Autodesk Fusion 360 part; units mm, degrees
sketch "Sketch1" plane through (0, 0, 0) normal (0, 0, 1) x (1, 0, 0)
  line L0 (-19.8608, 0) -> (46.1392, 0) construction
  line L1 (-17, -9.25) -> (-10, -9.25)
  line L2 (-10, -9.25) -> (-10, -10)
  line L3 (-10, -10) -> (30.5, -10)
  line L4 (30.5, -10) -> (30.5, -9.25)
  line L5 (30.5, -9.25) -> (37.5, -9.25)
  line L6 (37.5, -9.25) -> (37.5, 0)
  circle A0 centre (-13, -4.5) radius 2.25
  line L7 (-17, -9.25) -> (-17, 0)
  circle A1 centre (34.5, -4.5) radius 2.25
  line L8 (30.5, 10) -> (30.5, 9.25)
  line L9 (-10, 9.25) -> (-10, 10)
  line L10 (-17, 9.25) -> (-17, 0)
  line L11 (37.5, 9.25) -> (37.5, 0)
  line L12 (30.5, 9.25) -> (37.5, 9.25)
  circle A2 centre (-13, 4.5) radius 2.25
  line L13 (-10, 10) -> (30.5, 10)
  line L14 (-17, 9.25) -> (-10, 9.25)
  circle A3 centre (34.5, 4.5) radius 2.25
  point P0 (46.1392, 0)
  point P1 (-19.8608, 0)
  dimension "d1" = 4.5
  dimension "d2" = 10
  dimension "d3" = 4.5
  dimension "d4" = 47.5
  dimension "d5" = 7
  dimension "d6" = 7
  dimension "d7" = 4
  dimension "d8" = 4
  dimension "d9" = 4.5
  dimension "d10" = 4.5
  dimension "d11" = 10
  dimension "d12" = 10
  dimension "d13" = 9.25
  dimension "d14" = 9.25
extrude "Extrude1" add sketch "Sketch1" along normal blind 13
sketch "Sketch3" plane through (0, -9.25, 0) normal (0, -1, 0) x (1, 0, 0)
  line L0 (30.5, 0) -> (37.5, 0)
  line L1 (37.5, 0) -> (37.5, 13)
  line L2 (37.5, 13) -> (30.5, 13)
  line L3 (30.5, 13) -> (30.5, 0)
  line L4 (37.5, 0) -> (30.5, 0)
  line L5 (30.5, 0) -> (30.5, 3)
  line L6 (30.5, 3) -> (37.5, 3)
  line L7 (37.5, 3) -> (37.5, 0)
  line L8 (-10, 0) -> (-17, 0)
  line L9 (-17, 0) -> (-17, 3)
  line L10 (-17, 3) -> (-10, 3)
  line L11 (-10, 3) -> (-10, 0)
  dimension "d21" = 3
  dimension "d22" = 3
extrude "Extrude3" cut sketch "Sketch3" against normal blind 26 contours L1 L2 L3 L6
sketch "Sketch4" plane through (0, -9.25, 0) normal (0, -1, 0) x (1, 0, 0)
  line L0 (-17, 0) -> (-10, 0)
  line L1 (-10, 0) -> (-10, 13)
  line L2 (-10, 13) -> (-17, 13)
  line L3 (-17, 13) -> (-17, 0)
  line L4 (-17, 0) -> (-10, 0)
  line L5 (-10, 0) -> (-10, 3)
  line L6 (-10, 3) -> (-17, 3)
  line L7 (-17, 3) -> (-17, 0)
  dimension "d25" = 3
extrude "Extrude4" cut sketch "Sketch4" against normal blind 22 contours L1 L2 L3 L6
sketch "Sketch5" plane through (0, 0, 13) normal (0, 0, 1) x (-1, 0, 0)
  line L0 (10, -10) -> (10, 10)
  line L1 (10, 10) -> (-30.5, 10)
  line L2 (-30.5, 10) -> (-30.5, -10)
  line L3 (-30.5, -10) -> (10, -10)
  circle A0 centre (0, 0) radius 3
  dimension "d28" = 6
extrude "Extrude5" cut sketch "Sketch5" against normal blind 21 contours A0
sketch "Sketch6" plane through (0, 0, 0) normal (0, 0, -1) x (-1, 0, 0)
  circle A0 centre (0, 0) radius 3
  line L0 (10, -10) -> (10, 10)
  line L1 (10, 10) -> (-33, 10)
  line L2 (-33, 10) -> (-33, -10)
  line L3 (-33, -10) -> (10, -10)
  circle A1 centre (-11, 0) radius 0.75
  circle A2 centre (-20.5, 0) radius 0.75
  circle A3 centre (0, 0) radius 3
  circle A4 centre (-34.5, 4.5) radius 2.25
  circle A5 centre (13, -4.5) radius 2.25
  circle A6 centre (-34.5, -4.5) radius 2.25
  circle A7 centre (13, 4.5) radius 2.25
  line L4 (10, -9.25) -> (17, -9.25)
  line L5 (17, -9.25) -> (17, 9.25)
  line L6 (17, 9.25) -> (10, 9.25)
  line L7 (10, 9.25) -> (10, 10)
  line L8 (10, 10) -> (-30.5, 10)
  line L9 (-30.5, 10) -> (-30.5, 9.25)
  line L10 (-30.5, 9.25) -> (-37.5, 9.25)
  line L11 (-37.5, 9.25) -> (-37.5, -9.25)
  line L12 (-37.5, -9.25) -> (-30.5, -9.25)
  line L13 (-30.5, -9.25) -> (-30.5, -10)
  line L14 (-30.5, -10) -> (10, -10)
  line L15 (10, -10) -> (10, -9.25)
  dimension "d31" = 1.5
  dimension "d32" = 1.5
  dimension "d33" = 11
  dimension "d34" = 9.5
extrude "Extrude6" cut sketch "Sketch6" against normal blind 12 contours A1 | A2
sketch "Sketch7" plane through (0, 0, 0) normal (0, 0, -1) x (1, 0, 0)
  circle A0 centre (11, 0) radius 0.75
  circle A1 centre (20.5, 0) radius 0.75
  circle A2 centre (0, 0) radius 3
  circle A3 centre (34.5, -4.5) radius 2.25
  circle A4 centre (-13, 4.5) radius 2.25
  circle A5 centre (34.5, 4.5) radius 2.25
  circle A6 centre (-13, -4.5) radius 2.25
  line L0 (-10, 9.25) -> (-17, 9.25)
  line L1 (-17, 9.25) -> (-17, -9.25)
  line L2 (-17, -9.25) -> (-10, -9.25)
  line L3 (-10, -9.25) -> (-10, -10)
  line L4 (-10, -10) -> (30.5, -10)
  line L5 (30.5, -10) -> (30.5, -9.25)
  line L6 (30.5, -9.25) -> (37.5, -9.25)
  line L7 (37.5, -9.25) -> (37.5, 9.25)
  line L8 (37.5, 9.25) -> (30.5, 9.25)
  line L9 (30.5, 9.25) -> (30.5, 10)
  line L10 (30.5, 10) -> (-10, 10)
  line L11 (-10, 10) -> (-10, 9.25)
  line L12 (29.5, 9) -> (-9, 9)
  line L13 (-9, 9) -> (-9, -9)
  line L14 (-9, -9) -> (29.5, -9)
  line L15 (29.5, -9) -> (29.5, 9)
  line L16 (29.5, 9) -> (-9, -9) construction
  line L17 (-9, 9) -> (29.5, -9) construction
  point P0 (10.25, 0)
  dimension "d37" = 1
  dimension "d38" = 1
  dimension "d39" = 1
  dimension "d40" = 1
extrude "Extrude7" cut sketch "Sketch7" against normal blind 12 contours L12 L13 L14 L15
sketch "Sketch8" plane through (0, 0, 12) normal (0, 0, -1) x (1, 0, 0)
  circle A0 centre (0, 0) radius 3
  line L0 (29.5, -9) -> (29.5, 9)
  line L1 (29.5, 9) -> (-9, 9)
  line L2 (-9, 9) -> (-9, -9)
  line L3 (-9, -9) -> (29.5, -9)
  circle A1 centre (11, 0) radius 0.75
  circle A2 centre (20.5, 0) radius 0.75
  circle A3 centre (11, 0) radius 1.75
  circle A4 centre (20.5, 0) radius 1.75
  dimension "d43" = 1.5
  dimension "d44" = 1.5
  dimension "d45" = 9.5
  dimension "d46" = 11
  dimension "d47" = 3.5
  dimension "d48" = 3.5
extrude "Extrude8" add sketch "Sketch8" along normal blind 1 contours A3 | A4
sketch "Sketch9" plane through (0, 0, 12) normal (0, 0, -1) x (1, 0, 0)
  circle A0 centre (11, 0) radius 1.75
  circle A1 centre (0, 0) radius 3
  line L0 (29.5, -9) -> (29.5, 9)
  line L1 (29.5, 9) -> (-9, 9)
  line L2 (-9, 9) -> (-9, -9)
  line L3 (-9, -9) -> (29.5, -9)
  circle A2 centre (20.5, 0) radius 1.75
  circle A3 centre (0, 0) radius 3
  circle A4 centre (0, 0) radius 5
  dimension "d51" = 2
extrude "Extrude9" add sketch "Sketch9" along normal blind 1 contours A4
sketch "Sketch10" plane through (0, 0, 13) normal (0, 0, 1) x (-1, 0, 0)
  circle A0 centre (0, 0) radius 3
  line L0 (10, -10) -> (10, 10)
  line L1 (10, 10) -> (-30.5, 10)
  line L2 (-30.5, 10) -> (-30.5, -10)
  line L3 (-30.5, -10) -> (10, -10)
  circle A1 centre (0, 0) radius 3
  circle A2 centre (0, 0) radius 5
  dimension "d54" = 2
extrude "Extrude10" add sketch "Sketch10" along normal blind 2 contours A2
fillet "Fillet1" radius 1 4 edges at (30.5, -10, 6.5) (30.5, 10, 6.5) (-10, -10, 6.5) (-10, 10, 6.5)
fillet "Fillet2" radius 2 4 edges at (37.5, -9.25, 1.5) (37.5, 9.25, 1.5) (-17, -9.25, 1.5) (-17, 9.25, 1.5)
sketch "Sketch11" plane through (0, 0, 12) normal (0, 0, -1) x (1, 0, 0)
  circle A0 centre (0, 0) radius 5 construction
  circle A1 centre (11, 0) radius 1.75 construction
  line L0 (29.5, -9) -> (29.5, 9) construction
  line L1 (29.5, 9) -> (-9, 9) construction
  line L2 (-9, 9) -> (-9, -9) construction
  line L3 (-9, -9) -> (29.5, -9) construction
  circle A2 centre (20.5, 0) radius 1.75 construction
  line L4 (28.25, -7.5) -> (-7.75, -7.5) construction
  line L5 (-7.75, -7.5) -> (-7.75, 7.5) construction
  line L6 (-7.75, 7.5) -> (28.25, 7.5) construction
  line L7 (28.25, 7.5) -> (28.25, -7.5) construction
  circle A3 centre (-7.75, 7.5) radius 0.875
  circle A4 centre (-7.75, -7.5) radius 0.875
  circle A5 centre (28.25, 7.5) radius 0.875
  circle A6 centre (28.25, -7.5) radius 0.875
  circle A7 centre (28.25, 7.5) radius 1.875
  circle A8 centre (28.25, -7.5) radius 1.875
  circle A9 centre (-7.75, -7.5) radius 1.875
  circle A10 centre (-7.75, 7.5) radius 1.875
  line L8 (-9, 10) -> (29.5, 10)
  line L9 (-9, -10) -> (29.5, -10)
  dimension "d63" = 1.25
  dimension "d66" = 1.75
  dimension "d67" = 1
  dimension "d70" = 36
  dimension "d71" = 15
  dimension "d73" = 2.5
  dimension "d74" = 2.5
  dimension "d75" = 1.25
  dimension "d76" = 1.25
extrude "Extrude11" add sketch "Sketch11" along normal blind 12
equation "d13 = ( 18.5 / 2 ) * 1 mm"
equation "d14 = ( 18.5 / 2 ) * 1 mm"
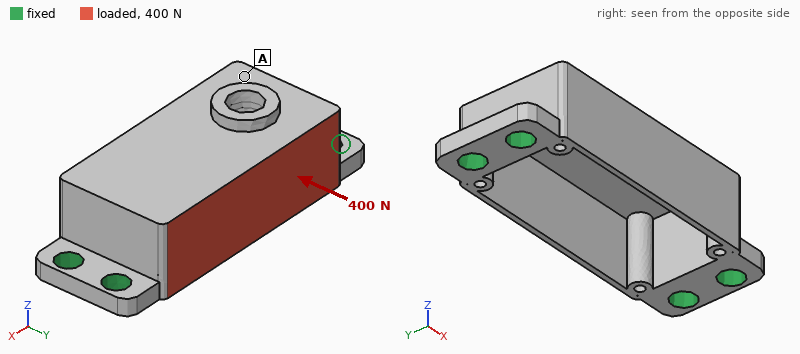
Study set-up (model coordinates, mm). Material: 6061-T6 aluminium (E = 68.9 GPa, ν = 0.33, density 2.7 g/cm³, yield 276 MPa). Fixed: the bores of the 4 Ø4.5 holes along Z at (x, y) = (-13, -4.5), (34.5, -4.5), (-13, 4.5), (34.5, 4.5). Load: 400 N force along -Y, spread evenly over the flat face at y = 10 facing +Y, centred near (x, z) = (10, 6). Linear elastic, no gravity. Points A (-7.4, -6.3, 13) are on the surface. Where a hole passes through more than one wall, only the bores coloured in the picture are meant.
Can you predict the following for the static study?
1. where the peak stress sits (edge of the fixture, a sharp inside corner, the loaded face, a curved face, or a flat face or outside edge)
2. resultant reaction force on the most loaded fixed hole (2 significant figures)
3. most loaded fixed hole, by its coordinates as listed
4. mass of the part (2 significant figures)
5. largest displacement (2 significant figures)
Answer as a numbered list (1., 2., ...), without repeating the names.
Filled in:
1. the loaded face
2. 170 N
3. (-13, 4.5)
4. 8.8 g
5. 0.29 mm
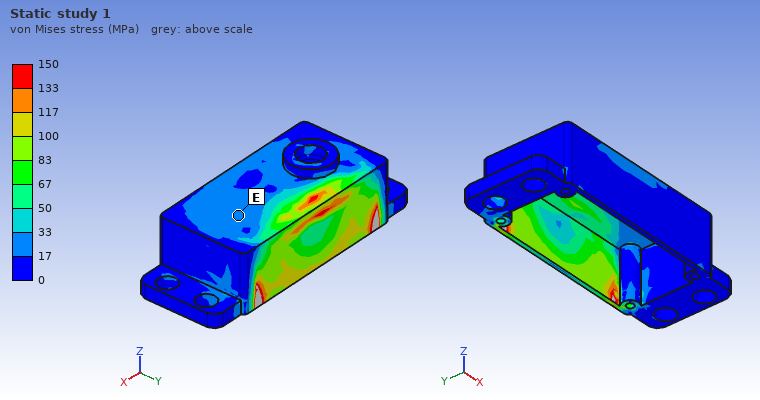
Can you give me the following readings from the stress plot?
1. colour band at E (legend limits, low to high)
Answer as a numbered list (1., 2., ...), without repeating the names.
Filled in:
1. 17 to 33 MPa
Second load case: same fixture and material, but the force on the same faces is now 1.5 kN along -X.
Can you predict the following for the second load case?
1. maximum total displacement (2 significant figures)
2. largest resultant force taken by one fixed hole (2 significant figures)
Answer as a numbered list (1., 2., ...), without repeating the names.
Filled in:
1. 35 µm
2. 640 N
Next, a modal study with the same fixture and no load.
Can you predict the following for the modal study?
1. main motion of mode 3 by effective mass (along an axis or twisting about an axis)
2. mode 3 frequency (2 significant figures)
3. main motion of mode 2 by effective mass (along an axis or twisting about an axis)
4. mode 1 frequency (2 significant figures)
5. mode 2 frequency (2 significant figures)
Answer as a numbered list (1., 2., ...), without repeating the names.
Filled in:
1. along Z
2. 13 kHz
3. along Y
4. 6500 Hz
5. 7200 Hz
